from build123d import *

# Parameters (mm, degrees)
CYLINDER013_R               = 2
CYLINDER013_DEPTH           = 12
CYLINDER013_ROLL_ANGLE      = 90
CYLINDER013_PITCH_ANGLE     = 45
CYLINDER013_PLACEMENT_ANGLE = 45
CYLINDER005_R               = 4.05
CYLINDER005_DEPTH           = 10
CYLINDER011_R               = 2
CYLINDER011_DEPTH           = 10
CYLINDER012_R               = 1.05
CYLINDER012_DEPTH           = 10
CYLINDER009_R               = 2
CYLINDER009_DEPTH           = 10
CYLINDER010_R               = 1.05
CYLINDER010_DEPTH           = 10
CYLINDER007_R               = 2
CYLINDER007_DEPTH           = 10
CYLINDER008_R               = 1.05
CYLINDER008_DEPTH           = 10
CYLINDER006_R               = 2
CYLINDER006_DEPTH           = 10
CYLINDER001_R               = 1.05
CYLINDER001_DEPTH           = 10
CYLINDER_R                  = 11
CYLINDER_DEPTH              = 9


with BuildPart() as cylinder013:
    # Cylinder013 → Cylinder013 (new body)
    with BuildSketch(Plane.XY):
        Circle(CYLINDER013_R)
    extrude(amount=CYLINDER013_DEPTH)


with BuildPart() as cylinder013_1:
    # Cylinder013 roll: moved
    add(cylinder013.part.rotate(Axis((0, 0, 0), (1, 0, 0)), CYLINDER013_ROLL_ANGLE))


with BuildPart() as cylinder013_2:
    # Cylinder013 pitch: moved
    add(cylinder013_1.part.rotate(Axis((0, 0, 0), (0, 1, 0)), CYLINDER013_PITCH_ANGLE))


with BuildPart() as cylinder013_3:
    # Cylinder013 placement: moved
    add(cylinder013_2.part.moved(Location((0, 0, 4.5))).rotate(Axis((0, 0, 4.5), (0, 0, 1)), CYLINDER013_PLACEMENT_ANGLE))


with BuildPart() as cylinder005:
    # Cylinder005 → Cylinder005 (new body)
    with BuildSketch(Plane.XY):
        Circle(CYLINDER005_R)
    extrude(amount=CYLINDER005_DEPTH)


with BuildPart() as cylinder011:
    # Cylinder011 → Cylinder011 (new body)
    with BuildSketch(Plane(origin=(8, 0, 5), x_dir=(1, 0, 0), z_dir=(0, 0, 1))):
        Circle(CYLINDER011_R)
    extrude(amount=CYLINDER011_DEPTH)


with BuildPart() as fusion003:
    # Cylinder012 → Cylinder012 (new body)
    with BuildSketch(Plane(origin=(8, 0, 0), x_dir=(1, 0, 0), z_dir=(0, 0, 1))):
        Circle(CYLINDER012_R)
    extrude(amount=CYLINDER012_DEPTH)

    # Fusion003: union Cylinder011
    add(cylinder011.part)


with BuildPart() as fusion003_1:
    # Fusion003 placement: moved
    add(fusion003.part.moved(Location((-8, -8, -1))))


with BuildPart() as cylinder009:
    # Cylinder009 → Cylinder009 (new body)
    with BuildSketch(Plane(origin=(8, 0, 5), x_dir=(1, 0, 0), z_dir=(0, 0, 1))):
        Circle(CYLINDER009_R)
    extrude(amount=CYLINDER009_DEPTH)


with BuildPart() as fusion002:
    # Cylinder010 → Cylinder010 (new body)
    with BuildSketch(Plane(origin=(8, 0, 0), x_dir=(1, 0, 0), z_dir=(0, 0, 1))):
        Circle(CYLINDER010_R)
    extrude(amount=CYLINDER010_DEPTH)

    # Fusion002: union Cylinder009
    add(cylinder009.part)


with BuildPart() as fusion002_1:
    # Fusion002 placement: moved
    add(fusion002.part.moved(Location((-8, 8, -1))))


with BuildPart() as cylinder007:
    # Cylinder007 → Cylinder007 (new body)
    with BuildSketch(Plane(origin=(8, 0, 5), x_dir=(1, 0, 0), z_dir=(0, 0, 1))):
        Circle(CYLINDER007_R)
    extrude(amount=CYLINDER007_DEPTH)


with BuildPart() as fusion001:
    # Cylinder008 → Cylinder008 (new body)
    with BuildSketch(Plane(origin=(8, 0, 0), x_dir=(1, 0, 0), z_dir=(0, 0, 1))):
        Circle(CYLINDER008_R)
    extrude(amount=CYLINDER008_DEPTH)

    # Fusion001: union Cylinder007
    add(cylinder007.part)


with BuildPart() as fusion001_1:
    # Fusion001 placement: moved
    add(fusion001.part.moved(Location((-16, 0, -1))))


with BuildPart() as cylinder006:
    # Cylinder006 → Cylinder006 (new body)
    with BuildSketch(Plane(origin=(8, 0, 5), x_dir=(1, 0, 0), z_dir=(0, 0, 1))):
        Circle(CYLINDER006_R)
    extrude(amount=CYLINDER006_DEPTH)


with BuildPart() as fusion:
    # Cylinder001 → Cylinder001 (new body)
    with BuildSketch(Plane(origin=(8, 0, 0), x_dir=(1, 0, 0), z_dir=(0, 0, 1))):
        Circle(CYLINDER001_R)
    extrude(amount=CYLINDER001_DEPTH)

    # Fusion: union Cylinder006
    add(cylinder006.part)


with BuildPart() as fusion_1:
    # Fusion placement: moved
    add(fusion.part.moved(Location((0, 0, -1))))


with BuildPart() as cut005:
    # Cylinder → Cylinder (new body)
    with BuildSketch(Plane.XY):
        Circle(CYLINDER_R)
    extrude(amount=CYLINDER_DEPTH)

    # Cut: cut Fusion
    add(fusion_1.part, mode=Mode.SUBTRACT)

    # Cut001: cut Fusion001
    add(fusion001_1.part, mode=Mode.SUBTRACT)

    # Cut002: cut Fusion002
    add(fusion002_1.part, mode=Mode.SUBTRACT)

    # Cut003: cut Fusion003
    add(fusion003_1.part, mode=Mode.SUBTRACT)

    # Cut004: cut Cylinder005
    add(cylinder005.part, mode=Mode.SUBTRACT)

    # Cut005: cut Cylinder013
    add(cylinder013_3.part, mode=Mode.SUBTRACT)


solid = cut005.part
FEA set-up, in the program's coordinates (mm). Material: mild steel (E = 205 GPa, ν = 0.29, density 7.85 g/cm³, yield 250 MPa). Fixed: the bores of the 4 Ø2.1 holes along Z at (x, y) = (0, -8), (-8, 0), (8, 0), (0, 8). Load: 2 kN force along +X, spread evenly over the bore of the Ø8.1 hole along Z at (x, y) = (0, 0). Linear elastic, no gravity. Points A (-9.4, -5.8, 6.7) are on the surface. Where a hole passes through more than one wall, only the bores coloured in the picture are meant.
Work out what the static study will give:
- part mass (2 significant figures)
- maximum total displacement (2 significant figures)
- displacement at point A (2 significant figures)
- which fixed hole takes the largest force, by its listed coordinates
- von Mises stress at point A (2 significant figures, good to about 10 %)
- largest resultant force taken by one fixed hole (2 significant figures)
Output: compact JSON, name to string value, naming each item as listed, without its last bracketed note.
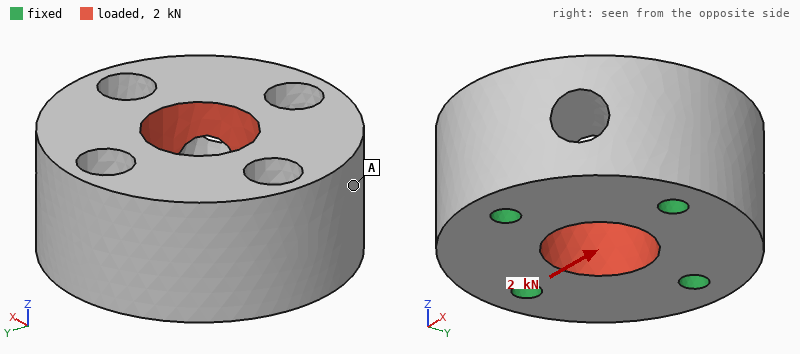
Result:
{"part mass": "20 g", "maximum total displacement": "1.4 µm", "displacement at point A": "0.86 µm", "which fixed hole takes the largest force, by its listed coordinates": "(-8, 0)", "von Mises stress at point A": "6.1 MPa", "largest resultant force taken by one fixed hole": "610 N"}
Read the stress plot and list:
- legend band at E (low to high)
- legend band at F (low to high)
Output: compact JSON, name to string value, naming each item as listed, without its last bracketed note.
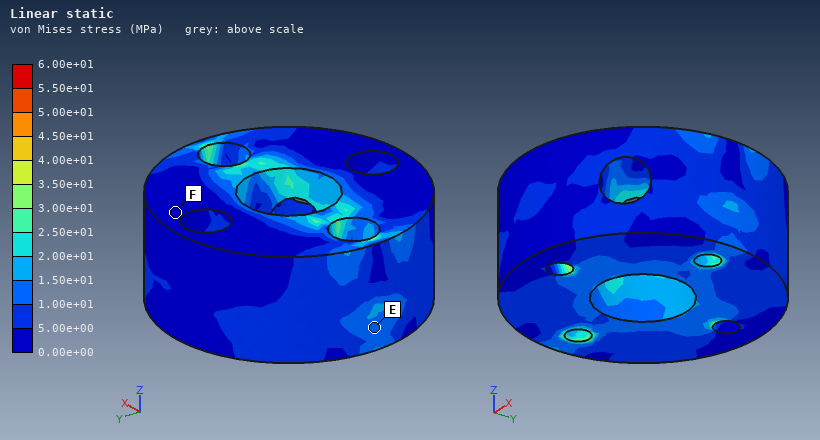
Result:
{"legend band at E": "1.00e+01 to 1.50e+01 MPa", "legend band at F": "0.00e+00 to 5.00e+00 MPa"}
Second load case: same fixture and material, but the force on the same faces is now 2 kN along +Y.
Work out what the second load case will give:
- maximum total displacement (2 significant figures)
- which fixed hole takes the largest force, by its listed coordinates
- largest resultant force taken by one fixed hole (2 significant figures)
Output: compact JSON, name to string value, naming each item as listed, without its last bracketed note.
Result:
{"maximum total displacement": "1.4 µm", "which fixed hole takes the largest force, by its listed coordinates": "(0, 8)", "largest resultant force taken by one fixed hole": "610 N"}
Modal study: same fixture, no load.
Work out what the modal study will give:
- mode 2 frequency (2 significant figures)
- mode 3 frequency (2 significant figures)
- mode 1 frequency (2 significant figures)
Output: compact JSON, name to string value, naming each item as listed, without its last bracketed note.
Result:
{"mode 2 frequency": "55 kHz", "mode 3 frequency": "59 kHz", "mode 1 frequency": "55 kHz"}
